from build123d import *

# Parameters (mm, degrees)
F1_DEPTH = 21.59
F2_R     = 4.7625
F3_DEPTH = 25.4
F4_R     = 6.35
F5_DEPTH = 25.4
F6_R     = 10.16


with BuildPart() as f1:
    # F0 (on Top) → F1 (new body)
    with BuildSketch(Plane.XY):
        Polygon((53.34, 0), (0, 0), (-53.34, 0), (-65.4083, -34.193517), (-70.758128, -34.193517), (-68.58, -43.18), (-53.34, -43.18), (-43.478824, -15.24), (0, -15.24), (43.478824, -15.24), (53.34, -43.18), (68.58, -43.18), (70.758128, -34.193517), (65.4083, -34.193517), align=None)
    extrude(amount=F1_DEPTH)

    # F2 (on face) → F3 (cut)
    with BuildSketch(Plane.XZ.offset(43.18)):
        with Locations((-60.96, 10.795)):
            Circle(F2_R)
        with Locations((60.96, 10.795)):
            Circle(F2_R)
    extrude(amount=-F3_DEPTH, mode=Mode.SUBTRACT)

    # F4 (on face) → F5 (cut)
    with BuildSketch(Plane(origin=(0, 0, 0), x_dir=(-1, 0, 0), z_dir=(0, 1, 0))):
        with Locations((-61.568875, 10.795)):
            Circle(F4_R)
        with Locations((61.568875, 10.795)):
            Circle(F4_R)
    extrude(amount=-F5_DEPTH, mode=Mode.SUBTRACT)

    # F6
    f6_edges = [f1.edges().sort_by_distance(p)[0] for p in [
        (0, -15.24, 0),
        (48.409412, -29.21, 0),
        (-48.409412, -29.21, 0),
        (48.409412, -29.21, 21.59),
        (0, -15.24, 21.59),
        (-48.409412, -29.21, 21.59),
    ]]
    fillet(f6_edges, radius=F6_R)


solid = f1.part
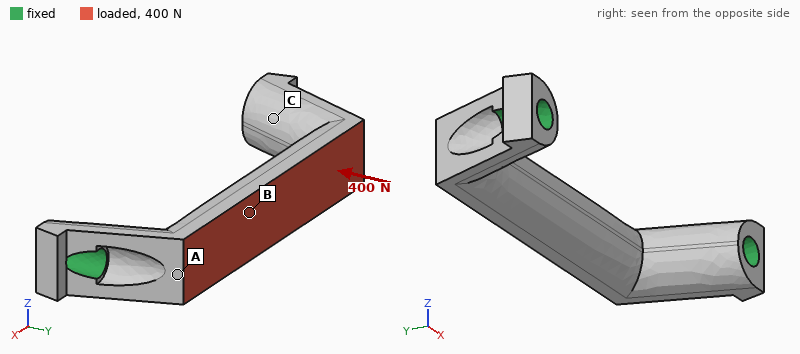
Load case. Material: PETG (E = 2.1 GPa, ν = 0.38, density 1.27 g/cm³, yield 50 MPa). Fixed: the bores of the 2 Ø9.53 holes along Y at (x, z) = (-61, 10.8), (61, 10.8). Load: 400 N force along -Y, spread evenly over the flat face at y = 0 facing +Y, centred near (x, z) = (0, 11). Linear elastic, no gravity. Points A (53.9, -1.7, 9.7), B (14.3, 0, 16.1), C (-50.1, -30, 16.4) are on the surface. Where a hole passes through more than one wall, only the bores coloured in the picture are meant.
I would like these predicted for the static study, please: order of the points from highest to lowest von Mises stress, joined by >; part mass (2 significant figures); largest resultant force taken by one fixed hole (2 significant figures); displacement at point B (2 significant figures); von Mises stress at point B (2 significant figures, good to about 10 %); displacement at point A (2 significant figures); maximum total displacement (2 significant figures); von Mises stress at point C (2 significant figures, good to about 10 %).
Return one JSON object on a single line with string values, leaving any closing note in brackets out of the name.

{"order of the points from highest to lowest von Mises stress, joined by >": "B > C > A", "part mass": "58 g", "largest resultant force taken by one fixed hole": "270 N", "displacement at point B": "0.15 mm", "von Mises stress at point B": "2.8 MPa", "displacement at point A": "0.027 mm", "maximum total displacement": "0.18 mm", "von Mises stress at point C": "1.1 MPa"}
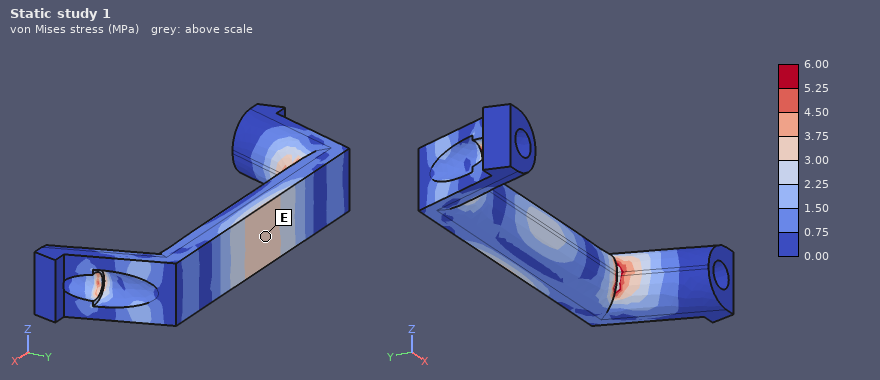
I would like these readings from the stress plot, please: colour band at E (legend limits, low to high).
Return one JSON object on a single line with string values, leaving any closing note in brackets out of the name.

{"colour band at E": "3.00 to 3.75 MPa"}
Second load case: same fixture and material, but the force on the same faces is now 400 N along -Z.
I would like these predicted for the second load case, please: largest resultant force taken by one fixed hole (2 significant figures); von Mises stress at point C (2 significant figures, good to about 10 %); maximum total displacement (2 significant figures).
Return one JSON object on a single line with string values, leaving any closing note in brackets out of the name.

{"largest resultant force taken by one fixed hole": "200 N", "von Mises stress at point C": "3.6 MPa", "maximum total displacement": "0.43 mm"}
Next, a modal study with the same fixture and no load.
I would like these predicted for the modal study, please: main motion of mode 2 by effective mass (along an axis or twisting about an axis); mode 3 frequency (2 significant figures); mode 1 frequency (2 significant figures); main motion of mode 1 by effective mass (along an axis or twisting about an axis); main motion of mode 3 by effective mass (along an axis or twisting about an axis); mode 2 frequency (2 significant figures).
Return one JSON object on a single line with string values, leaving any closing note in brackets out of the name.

{"main motion of mode 2 by effective mass": "along Y", "mode 3 frequency": "1500 Hz", "mode 1 frequency": "1000 Hz", "main motion of mode 1 by effective mass": "along Z", "main motion of mode 3 by effective mass": "along X", "mode 2 frequency": "1400 Hz"}
